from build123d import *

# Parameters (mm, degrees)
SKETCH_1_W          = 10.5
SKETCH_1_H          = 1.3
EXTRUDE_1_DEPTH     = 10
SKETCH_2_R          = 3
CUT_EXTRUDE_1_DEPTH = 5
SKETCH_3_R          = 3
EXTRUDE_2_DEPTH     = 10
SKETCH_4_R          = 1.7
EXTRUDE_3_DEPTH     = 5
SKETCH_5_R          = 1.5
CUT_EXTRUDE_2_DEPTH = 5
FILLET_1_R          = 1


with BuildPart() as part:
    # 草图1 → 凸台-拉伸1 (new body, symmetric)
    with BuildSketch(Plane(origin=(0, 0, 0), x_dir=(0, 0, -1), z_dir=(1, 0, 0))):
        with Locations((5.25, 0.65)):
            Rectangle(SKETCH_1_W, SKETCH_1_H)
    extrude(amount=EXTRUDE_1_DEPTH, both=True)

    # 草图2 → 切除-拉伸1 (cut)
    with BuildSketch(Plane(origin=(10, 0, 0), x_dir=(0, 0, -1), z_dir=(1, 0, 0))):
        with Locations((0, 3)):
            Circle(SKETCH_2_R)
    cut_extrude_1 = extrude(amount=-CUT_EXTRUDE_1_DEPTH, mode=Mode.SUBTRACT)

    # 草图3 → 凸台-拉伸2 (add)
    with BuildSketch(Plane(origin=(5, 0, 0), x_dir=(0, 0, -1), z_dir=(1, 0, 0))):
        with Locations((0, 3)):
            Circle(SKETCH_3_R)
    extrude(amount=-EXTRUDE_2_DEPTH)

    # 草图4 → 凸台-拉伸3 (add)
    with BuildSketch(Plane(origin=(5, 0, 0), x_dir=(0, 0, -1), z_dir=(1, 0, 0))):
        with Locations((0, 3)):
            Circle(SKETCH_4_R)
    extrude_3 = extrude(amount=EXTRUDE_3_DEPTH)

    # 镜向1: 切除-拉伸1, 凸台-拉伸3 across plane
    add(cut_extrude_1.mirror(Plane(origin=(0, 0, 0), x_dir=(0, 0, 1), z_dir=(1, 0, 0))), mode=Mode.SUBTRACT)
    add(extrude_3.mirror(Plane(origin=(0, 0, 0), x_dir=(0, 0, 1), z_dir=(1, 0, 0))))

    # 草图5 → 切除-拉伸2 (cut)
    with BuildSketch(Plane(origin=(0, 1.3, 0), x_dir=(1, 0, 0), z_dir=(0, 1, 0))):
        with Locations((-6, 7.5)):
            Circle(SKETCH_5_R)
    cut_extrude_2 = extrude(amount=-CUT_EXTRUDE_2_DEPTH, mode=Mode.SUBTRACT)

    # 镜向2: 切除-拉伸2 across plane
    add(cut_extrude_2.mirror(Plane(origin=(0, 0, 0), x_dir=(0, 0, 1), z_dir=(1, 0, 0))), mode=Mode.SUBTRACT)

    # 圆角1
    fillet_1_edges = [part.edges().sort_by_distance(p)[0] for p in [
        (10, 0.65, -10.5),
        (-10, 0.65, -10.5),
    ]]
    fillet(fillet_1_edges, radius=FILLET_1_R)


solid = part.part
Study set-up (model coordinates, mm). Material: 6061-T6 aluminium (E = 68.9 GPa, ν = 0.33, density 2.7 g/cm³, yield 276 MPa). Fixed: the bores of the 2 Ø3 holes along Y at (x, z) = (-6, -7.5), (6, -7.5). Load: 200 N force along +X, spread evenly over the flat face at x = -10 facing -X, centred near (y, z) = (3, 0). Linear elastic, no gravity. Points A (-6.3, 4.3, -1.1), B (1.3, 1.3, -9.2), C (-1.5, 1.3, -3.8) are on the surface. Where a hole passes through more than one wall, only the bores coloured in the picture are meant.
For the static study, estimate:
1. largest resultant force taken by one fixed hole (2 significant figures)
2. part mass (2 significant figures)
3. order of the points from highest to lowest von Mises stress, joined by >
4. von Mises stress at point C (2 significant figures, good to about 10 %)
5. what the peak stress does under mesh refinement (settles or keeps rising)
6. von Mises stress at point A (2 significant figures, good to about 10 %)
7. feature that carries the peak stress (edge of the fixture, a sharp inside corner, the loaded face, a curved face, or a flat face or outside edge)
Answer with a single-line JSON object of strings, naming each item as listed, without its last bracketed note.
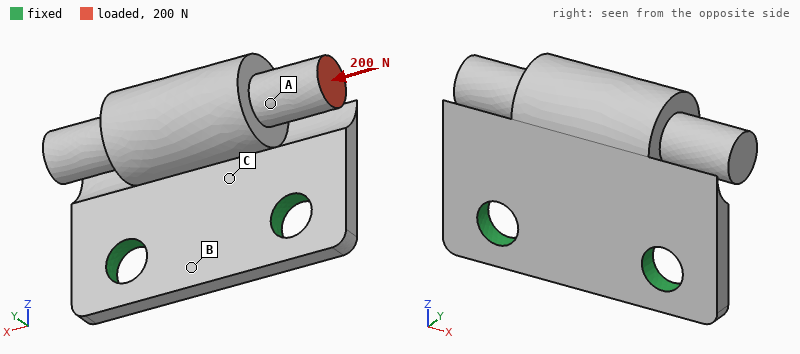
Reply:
{"largest resultant force taken by one fixed hole": "150 N", "part mass": "1.6 g", "order of the points from highest to lowest von Mises stress, joined by >": "C > A > B", "von Mises stress at point C": "39 MPa", "what the peak stress does under mesh refinement": "keeps rising", "von Mises stress at point A": "21 MPa", "feature that carries the peak stress": "a sharp inside corner"}
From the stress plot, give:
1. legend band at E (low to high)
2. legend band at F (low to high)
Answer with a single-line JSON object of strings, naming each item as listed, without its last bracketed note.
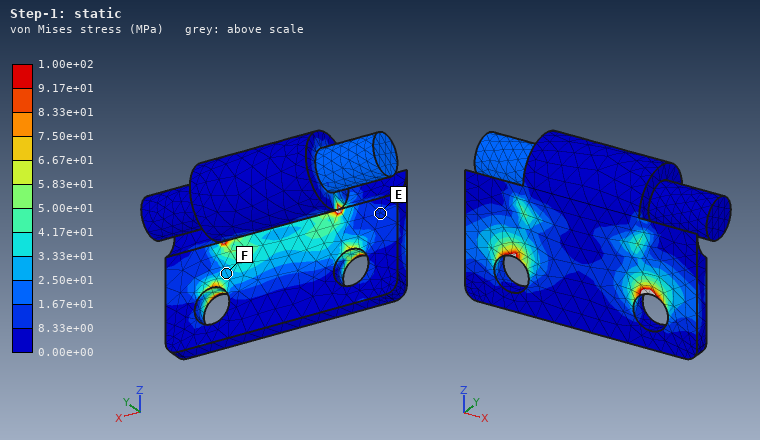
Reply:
{"legend band at E": "8.33e+00 to 1.67e+01 MPa", "legend band at F": "2.50e+01 to 3.33e+01 MPa"}
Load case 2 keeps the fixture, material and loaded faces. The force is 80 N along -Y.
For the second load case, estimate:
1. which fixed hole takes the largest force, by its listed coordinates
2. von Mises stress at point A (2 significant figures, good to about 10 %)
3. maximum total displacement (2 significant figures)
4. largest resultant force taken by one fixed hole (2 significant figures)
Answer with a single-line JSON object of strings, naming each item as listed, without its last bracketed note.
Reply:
{"which fixed hole takes the largest force, by its listed coordinates": "(-6, -7.5)", "von Mises stress at point A": "58 MPa", "maximum total displacement": "0.10 mm", "largest resultant force taken by one fixed hole": "120 N"}
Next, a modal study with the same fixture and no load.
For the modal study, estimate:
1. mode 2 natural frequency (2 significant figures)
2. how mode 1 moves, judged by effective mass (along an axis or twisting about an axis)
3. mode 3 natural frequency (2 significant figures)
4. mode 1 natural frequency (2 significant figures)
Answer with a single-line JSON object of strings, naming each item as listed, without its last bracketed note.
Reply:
{"mode 2 natural frequency": "15 kHz", "how mode 1 moves, judged by effective mass": "along Y", "mode 3 natural frequency": "26 kHz", "mode 1 natural frequency": "5900 Hz"}
